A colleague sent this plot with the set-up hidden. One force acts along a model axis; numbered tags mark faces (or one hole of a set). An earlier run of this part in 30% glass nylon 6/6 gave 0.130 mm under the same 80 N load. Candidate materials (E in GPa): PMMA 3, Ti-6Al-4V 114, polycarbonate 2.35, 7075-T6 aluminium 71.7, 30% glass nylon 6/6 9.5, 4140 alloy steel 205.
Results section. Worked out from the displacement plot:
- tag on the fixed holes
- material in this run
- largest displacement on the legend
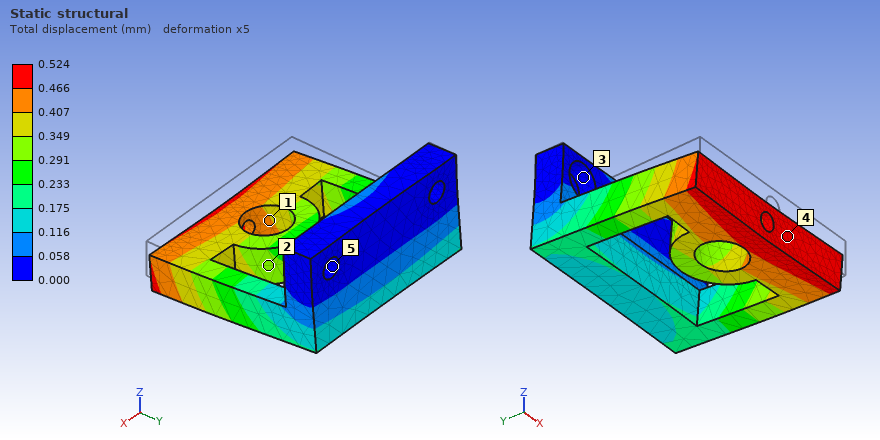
5
polycarbonate
0.524 mm
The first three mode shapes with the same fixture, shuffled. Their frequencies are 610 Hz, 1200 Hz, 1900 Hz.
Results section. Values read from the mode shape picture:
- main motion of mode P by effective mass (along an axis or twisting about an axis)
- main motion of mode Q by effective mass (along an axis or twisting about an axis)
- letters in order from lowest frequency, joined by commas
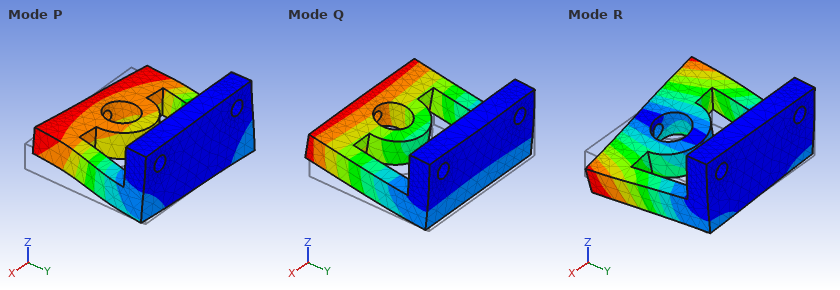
along X
along Z
Q, P, R
